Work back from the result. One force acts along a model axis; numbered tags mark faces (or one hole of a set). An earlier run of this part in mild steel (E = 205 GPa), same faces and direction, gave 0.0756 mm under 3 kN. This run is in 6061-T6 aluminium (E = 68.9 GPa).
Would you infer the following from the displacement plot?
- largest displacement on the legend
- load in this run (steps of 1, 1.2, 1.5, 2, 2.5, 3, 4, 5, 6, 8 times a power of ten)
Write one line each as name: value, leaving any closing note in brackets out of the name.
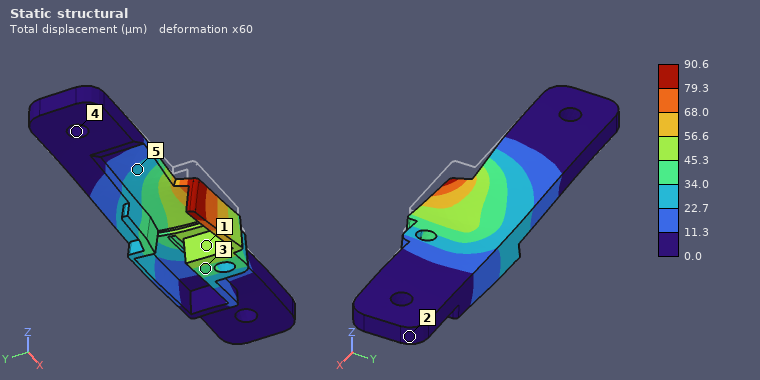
largest displacement on the legend: 90.6 µm
load in this run: 1.2 kN
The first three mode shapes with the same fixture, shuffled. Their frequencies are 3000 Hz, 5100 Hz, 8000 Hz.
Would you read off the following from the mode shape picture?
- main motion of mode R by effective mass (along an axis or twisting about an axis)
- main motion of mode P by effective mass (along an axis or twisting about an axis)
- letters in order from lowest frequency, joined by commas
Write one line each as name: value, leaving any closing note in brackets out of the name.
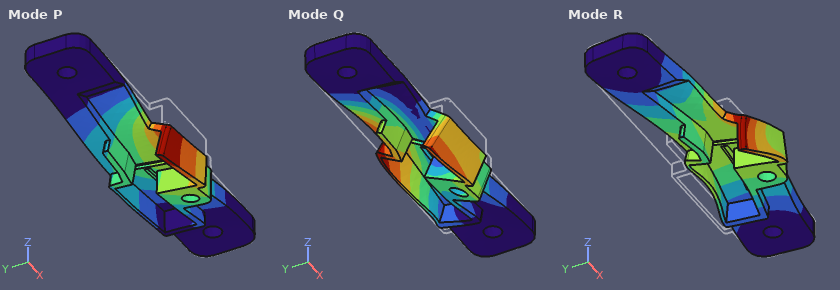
main motion of mode R by effective mass: along Y
main motion of mode P by effective mass: along Z
letters in order from lowest frequency, joined by commas: P, Q, R
